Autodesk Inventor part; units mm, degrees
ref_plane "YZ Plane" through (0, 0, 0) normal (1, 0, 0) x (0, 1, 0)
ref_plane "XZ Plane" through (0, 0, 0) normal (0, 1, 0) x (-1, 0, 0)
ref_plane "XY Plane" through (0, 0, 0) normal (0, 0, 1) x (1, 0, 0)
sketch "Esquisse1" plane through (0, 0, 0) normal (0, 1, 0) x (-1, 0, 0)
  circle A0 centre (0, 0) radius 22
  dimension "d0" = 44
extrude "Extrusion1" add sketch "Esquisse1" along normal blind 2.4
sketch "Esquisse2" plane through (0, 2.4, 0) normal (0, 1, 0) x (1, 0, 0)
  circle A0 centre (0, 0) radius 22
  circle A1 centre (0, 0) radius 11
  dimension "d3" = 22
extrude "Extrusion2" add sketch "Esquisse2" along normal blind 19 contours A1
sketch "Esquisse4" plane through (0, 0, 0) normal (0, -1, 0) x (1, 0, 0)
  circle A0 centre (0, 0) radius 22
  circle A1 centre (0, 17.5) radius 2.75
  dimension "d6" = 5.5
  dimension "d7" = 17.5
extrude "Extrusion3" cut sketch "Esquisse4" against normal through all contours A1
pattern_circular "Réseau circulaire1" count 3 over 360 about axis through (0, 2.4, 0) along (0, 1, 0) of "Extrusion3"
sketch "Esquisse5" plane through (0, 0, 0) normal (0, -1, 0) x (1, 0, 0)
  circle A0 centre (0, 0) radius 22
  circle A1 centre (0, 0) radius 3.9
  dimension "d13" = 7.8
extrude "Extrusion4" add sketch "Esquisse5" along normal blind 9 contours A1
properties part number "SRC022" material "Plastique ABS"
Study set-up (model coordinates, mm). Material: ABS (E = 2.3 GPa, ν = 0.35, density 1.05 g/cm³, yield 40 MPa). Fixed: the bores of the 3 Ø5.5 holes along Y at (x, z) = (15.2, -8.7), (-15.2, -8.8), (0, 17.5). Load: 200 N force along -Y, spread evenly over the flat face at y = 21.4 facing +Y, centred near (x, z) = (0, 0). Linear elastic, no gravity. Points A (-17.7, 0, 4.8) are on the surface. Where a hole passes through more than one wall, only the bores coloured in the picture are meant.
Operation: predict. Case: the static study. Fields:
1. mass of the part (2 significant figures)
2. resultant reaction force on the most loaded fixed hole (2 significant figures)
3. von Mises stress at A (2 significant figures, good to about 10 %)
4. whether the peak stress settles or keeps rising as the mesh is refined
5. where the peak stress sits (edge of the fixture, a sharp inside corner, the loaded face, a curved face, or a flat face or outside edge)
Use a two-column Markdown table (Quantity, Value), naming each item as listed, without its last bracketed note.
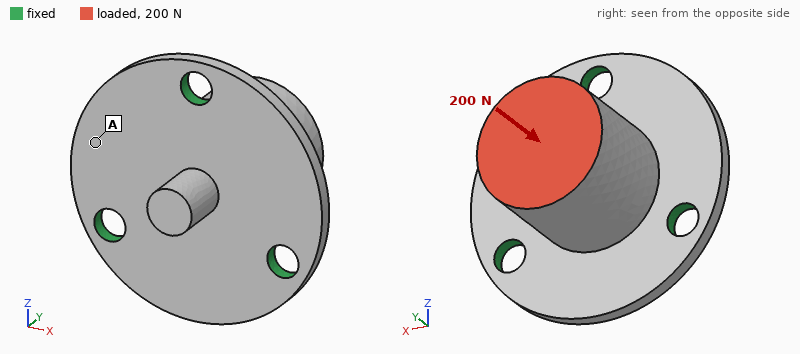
| Quantity | Value |
|---|---|
| mass of the part | 12 g |
| resultant reaction force on the most loaded fixed hole | 72 N |
| von Mises stress at A | 1.6 MPa |
| whether the peak stress settles or keeps rising as the mesh is refined | keeps rising |
| where the peak stress sits | edge of the fixture |
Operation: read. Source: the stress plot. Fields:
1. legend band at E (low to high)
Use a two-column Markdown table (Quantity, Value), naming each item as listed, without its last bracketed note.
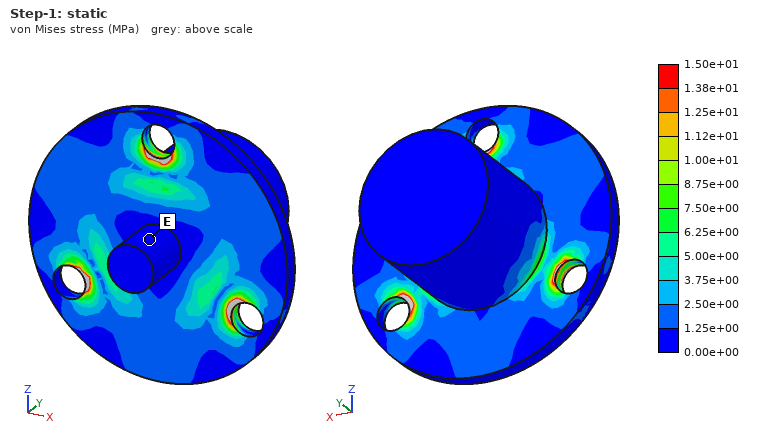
| Quantity | Value |
|---|---|
| legend band at E | 0.00e+00 to 1.25e+00 MPa |
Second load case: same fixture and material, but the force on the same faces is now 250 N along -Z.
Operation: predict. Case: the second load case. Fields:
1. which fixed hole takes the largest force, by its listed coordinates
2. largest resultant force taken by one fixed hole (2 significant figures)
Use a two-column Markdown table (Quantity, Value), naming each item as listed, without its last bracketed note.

| Quantity | Value |
|---|---|
| which fixed hole takes the largest force, by its listed coordinates | (0, 17.5) |
| largest resultant force taken by one fixed hole | 270 N |
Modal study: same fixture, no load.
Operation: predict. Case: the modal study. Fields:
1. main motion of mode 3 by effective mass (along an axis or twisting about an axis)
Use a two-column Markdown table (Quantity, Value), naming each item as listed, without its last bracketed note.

| Quantity | Value |
|---|---|
| main motion of mode 3 by effective mass | along Y |
